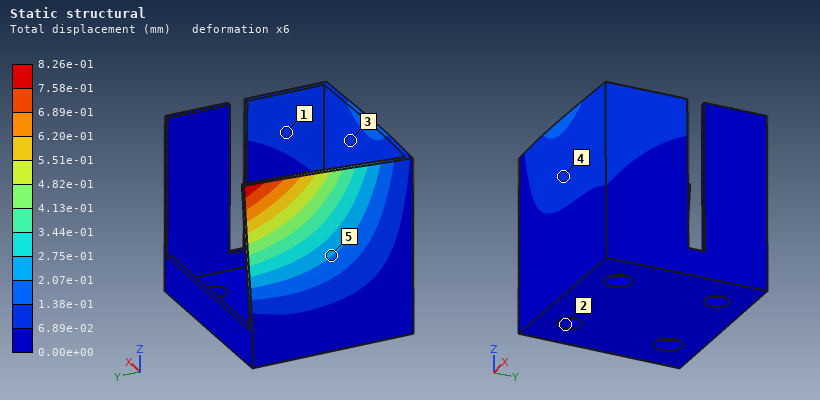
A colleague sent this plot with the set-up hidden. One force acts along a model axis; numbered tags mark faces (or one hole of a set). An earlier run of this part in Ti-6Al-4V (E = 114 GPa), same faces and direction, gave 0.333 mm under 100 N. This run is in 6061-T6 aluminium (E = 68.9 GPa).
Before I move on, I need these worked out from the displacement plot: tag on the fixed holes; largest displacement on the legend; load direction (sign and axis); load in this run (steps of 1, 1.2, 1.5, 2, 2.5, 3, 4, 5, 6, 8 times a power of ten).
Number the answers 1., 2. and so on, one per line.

1. 2
2. 8.26e-01 mm
3. +X
4. 150 N
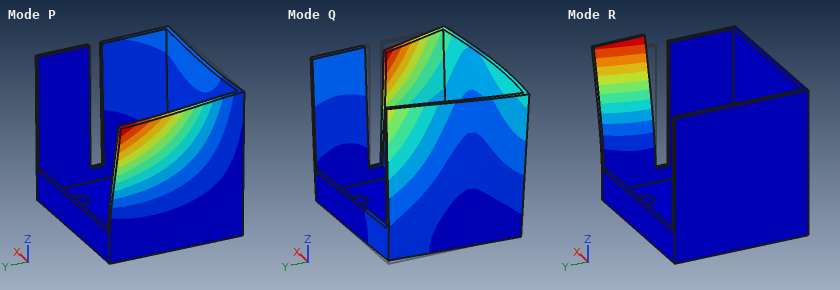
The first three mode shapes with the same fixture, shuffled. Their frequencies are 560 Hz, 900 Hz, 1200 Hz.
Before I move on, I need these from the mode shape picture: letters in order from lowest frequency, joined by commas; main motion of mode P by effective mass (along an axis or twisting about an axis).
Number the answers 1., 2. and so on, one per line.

1. R, P, Q
2. along X
